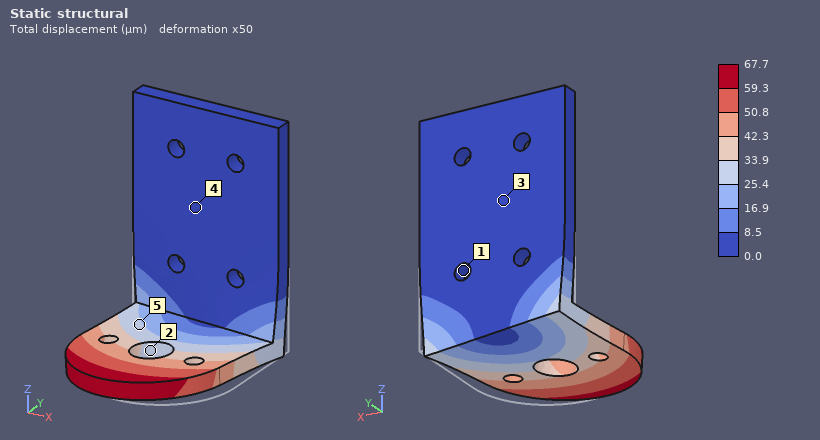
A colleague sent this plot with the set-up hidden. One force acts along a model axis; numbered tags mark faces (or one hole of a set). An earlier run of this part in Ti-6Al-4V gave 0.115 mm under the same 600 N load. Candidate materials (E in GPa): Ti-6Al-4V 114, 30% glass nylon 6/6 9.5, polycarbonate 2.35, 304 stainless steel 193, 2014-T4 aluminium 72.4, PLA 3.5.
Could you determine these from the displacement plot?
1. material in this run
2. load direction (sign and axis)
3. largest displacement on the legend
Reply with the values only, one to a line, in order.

304 stainless steel
-X
67.7 µm
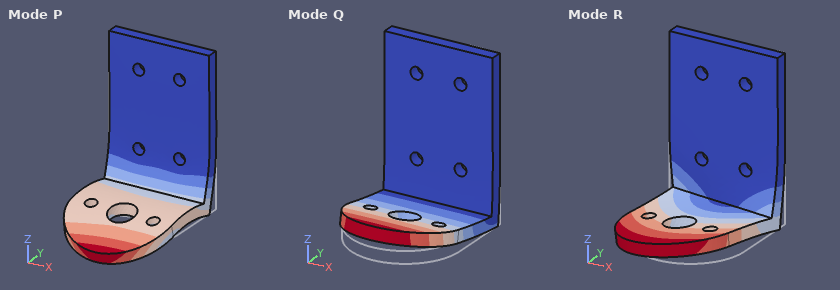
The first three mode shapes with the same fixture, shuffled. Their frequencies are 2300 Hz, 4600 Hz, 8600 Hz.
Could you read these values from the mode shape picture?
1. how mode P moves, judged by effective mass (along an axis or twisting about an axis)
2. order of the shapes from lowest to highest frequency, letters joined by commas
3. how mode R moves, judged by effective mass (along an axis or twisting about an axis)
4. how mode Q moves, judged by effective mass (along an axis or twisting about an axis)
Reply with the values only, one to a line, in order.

along Y
Q, R, P
along X
along Z
